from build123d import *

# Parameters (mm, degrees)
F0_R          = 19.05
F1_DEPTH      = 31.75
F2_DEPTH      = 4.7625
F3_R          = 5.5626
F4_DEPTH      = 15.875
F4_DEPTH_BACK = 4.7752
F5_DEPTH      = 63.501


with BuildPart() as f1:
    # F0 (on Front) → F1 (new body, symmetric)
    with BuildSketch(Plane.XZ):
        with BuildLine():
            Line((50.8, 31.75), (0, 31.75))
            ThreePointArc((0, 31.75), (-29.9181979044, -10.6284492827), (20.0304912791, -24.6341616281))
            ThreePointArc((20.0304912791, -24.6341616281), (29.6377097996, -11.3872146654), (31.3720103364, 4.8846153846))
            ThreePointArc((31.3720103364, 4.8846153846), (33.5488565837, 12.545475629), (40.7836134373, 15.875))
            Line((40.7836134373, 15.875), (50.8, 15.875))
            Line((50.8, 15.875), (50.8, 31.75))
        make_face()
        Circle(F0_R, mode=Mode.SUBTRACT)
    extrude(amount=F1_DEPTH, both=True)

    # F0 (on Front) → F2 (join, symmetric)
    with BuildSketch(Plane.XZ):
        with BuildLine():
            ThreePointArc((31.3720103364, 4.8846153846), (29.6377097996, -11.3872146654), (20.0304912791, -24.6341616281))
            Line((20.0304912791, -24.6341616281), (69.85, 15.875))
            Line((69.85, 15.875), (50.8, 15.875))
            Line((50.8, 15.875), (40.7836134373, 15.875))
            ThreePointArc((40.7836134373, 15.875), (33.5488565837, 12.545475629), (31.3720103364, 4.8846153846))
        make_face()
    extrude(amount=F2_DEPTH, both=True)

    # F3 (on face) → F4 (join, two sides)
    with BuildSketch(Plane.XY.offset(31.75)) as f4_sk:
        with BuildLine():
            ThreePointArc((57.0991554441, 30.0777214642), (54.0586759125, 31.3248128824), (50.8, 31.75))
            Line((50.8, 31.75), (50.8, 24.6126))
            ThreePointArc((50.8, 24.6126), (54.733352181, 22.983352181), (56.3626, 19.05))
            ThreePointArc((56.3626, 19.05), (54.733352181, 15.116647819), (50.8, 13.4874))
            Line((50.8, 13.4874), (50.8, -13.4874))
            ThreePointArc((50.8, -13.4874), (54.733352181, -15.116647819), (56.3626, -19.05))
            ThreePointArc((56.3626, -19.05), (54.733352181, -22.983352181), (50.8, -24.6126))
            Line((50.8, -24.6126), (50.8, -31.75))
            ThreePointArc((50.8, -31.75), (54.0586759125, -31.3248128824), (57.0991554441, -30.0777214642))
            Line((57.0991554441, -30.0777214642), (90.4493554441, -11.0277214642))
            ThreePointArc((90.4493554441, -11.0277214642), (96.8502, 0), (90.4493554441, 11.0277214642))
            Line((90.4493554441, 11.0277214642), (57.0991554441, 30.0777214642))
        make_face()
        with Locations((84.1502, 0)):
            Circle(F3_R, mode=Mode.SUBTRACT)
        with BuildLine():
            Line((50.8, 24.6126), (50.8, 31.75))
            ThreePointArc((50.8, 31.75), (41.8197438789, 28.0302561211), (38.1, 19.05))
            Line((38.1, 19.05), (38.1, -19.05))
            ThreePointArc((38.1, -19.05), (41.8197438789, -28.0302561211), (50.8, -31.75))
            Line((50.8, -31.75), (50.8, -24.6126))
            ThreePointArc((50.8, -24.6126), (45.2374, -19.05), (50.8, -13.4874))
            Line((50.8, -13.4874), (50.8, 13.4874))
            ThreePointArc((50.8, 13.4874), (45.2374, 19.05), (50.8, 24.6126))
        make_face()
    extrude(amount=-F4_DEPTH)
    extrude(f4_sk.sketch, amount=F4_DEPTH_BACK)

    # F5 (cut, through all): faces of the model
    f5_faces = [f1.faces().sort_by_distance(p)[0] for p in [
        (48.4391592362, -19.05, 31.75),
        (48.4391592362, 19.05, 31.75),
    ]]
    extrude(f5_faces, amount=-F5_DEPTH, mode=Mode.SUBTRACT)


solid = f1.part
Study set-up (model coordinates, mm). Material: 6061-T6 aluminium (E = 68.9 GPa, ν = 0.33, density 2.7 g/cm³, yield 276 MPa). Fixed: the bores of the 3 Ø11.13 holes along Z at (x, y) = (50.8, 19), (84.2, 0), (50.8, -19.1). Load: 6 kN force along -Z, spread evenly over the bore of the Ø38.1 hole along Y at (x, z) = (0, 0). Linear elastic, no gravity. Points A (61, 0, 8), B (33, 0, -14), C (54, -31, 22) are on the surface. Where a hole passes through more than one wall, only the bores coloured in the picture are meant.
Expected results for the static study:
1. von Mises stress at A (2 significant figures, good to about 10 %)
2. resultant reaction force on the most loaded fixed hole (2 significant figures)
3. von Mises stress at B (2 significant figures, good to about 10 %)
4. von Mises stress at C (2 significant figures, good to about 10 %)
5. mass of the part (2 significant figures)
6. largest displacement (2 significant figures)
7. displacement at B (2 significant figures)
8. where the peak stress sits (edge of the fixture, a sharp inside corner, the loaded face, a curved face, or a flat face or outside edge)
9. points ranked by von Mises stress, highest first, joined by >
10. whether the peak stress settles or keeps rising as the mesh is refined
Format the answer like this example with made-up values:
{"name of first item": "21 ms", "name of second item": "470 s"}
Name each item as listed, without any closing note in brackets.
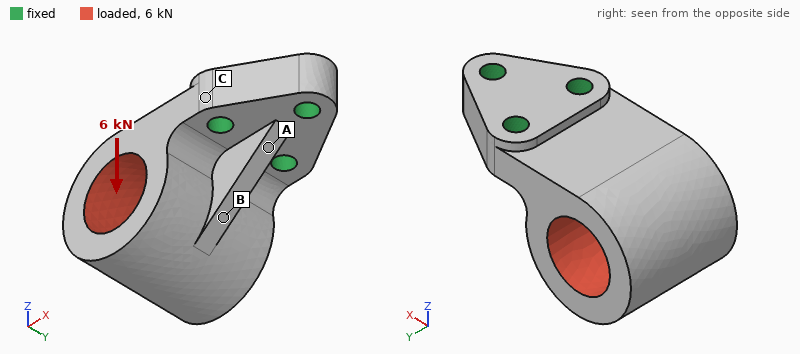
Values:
{"von Mises stress at A": "51 MPa", "resultant reaction force on the most loaded fixed hole": "4.3 kN", "von Mises stress at B": "28 MPa", "von Mises stress at C": "10 MPa", "mass of the part": "550 g", "largest displacement": "0.15 mm", "displacement at B": "0.060 mm", "where the peak stress sits": "edge of the fixture", "points ranked by von Mises stress, highest first, joined by >": "A > B > C", "whether the peak stress settles or keeps rising as the mesh is refined": "keeps rising"}
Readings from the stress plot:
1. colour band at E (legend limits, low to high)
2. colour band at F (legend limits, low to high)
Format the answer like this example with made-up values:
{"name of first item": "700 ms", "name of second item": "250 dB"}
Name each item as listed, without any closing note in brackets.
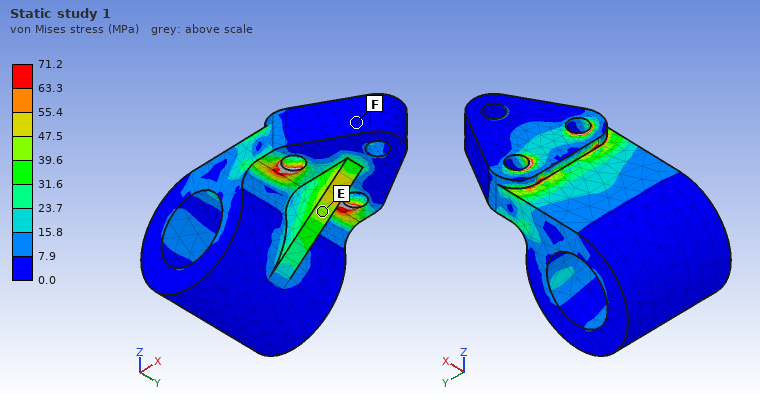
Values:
{"colour band at E": "39.6 to 47.5 MPa", "colour band at F": "0.0 to 7.9 MPa"}
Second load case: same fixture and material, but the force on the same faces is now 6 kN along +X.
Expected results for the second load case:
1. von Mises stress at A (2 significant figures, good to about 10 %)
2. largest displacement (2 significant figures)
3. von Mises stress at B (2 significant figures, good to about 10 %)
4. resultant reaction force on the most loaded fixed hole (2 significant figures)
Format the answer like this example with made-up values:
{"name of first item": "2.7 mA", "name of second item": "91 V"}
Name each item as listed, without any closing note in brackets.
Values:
{"von Mises stress at A": "33 MPa", "largest displacement": "82 µm", "von Mises stress at B": "24 MPa", "resultant reaction force on the most loaded fixed hole": "2.4 kN"}
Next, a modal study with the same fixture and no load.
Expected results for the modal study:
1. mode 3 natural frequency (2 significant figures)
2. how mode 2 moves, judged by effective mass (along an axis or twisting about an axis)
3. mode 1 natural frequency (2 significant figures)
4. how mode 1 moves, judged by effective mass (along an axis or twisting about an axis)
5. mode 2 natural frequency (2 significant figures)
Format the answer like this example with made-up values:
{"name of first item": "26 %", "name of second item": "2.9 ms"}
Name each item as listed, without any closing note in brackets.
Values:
{"mode 3 natural frequency": "5400 Hz", "how mode 2 moves, judged by effective mass": "along Y", "mode 1 natural frequency": "1800 Hz", "how mode 1 moves, judged by effective mass": "along Z", "mode 2 natural frequency": "3300 Hz"}
